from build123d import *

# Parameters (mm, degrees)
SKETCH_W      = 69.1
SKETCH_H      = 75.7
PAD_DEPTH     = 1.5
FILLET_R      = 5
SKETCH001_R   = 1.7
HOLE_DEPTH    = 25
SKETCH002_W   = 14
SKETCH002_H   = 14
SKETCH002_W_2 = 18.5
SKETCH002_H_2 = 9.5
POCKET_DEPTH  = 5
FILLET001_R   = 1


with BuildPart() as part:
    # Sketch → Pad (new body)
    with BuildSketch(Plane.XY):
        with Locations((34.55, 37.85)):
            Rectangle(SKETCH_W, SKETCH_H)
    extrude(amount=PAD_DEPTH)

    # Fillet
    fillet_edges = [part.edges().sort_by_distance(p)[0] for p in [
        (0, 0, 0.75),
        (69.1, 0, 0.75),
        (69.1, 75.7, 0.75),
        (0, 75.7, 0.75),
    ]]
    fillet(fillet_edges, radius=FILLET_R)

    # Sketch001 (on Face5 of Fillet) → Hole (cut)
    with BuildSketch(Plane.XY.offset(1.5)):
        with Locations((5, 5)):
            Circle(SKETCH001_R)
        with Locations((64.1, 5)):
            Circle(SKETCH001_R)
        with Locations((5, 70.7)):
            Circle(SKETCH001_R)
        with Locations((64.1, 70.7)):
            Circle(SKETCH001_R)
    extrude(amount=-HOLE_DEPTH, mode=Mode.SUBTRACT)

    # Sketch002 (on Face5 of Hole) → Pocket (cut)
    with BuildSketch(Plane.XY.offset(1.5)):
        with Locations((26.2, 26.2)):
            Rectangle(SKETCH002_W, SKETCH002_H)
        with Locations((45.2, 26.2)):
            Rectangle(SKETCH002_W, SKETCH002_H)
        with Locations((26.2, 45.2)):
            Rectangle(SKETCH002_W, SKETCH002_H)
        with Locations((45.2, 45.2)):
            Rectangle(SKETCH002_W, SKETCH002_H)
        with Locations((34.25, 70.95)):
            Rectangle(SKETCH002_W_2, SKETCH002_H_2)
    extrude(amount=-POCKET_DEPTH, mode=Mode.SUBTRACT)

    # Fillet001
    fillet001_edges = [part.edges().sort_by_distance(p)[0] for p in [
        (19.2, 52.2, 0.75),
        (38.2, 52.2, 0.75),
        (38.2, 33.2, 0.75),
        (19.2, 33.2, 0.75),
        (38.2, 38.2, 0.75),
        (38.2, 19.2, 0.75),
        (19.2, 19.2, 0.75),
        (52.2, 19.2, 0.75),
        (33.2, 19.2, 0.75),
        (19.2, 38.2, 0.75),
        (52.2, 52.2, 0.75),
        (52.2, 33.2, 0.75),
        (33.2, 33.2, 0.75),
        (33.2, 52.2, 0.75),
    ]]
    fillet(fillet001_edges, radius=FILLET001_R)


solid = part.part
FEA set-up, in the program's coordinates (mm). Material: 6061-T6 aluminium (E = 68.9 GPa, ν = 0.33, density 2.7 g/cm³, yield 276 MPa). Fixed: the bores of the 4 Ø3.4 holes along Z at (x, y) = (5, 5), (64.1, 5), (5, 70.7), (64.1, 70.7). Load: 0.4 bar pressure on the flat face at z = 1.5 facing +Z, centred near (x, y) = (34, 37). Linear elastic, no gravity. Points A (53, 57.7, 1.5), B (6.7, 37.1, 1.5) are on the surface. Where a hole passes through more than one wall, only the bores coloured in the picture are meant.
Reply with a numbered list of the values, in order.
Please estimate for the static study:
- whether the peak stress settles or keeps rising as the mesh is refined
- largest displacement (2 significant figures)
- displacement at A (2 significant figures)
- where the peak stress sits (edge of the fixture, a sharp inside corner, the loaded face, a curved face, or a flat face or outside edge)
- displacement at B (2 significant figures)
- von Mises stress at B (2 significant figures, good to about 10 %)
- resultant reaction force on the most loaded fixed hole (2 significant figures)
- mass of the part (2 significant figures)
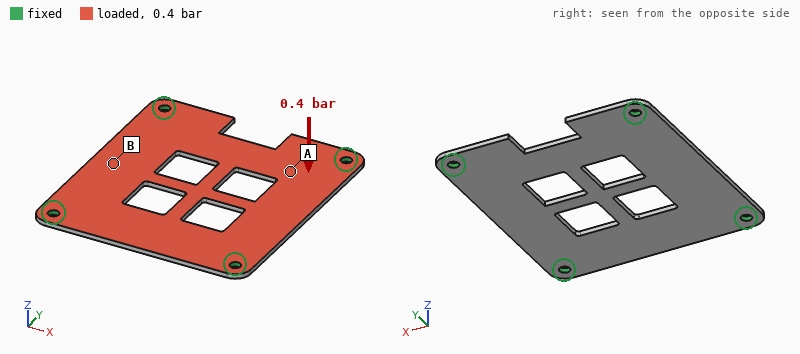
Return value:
1. keeps rising
2. 0.23 mm
3. 0.097 mm
4. edge of the fixture
5. 0.13 mm
6. 22 MPa
7. 44 N
8. 17 g
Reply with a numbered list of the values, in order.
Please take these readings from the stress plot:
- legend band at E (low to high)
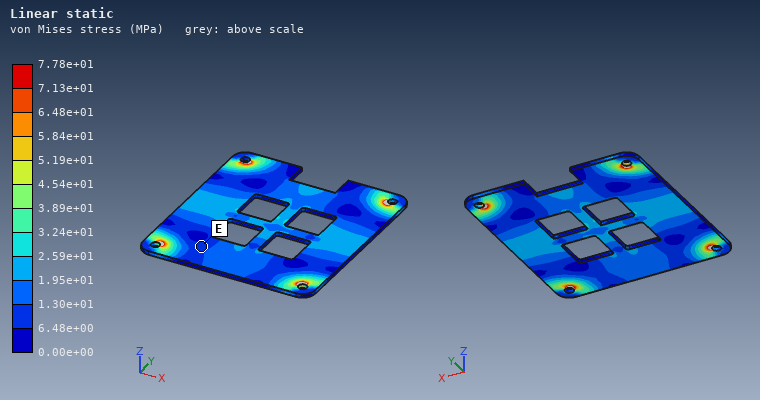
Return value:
1. 6.48e+00 to 1.30e+01 MPa
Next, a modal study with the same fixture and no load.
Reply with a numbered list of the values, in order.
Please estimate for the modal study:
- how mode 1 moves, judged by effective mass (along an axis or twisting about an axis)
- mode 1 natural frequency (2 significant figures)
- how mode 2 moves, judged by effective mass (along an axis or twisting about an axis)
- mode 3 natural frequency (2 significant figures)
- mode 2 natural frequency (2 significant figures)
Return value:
1. along Z
2. 1400 Hz
3. twisting about Y
4. 2400 Hz
5. 2100 Hz
